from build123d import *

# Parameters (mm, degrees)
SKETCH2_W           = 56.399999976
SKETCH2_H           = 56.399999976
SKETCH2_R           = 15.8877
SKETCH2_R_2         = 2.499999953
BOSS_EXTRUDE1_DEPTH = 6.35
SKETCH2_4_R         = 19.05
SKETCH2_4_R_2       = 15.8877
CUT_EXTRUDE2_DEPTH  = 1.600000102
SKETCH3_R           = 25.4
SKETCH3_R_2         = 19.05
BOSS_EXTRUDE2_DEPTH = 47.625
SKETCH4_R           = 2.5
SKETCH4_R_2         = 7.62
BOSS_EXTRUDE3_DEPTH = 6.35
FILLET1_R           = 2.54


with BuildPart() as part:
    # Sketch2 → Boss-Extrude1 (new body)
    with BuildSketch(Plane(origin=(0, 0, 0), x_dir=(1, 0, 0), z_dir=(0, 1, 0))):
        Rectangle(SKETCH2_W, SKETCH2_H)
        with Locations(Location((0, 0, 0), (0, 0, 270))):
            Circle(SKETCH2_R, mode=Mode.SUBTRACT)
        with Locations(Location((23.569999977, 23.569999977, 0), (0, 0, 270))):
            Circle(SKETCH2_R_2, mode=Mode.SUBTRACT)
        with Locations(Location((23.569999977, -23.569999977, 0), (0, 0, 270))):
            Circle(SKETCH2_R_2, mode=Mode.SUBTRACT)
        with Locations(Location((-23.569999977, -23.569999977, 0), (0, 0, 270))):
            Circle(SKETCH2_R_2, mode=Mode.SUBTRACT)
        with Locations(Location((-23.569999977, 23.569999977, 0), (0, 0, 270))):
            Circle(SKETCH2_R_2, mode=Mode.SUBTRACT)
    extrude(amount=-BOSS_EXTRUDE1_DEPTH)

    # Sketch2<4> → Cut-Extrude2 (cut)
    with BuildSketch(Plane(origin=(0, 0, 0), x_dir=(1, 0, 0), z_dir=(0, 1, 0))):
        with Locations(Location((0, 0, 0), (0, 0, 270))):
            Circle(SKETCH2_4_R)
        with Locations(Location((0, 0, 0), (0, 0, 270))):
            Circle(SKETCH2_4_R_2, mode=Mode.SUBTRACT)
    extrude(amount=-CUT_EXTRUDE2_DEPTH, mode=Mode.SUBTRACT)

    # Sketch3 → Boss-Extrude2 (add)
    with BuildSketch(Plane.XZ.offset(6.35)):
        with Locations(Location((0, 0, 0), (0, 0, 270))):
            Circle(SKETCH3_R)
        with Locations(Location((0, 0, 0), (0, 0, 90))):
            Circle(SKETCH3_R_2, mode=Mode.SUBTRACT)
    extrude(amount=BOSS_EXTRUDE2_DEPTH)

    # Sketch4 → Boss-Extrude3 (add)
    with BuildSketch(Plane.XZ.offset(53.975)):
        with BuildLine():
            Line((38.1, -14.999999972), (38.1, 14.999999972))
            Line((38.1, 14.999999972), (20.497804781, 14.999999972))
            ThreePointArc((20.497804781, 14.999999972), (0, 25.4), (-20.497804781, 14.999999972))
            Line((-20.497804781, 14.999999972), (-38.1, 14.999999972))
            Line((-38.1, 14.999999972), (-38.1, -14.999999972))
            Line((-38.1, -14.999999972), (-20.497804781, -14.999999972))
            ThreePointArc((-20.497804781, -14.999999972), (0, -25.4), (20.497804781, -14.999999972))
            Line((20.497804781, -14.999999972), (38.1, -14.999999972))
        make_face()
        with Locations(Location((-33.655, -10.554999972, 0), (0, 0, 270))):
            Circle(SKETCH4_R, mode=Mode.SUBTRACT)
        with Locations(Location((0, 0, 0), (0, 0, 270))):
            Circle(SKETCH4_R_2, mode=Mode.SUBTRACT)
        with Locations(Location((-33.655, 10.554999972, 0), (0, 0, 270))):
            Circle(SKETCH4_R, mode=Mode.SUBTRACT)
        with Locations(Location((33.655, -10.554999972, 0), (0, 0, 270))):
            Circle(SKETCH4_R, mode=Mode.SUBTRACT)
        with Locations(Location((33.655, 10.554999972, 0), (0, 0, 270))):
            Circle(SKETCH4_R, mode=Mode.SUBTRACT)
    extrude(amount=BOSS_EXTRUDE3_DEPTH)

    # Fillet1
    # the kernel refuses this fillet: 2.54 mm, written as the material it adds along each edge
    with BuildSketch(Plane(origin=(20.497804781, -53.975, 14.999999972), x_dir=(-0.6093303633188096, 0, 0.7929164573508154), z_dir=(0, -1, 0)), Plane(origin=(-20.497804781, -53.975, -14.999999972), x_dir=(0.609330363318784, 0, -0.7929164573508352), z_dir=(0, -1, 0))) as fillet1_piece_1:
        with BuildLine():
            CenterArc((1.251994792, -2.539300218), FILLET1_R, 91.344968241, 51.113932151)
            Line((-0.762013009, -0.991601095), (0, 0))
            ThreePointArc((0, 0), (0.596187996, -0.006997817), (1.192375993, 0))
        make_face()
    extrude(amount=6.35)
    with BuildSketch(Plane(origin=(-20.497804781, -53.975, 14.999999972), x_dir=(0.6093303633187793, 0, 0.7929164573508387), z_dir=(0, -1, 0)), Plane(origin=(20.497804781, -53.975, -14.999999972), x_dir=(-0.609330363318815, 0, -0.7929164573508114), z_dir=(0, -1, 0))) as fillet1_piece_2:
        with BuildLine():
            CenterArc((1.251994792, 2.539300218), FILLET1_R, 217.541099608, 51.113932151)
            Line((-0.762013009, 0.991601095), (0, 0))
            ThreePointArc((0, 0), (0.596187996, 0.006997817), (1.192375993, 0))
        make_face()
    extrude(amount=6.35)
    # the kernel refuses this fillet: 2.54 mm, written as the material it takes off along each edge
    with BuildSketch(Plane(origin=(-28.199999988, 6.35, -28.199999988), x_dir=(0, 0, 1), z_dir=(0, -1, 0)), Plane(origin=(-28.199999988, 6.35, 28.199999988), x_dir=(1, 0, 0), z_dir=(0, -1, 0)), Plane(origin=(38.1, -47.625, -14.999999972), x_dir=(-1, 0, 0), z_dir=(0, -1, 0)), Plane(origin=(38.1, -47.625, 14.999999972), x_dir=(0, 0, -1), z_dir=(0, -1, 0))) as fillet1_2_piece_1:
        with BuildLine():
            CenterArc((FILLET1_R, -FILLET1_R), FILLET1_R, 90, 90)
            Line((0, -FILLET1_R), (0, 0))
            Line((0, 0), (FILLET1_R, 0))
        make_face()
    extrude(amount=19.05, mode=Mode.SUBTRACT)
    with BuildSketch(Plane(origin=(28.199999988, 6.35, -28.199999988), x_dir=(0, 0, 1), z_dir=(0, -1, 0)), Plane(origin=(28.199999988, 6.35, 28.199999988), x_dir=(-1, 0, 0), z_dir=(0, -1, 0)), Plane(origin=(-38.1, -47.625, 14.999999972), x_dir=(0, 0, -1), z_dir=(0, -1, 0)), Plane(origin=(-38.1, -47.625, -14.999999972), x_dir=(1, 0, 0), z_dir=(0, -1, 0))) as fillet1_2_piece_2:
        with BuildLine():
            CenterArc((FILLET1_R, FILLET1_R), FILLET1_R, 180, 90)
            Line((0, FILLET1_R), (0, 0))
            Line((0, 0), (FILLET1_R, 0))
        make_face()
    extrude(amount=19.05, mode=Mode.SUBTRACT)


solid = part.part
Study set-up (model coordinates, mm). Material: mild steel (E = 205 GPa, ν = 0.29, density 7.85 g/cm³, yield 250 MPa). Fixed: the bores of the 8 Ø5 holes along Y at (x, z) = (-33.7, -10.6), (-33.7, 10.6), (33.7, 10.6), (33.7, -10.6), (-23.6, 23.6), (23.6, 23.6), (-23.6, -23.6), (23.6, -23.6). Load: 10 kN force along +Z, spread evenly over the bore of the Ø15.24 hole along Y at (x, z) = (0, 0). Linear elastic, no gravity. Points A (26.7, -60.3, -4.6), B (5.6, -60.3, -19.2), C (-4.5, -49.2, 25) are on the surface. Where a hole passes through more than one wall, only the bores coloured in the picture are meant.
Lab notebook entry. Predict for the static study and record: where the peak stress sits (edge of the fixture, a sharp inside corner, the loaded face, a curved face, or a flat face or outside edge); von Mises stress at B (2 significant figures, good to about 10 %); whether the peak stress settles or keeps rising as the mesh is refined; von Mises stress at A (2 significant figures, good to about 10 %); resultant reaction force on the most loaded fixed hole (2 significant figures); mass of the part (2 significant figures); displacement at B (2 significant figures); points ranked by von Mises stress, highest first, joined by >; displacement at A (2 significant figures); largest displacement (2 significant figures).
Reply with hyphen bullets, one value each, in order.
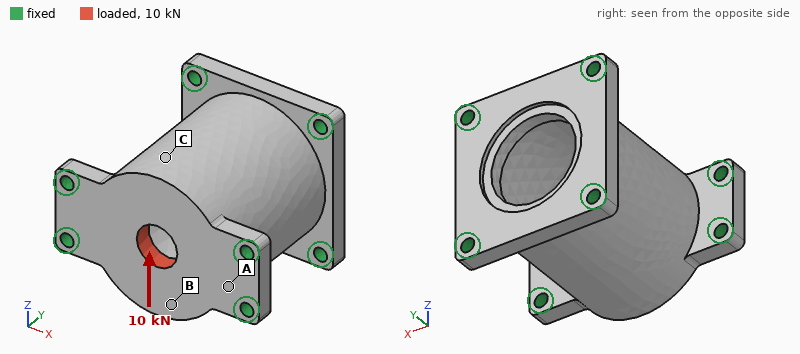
- edge of the fixture
- 27 MPa
- keeps rising
- 56 MPa
- 3.0 kN
- 570 g
- 8.8 µm
- A > B > C
- 2.4 µm
- 10 µm
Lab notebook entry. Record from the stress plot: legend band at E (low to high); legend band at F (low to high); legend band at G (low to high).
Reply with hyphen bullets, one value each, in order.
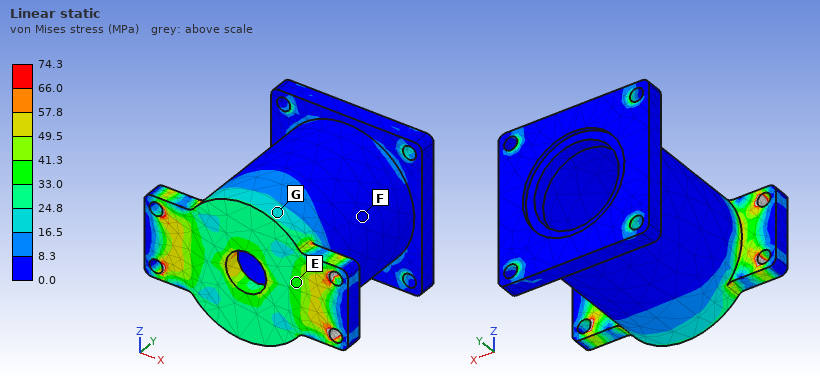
- 33.0 to 41.3 MPa
- 0.0 to 8.3 MPa
- 16.5 to 24.8 MPa
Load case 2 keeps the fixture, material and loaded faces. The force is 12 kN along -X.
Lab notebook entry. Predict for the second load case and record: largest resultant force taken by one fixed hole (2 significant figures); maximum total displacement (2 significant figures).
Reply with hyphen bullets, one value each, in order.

- 2.9 kN
- 5.3 µm
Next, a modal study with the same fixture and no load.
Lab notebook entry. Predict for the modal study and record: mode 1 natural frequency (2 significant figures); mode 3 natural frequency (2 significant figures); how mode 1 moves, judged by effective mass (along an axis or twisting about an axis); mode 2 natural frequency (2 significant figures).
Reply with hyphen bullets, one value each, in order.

- 9600 Hz
- 13 kHz
- along Y
- 13 kHz
